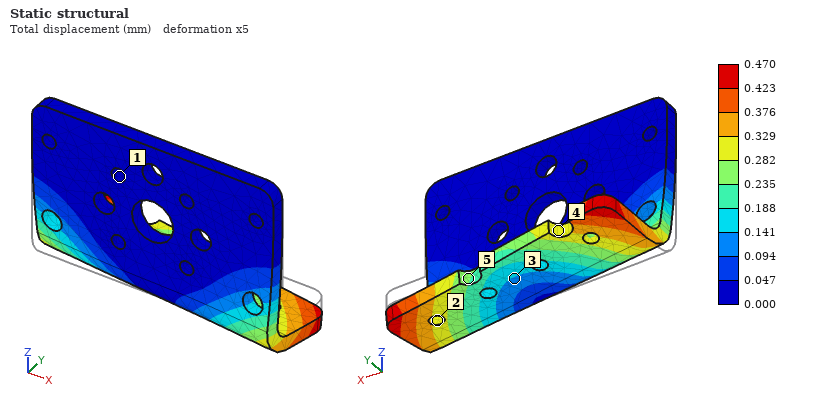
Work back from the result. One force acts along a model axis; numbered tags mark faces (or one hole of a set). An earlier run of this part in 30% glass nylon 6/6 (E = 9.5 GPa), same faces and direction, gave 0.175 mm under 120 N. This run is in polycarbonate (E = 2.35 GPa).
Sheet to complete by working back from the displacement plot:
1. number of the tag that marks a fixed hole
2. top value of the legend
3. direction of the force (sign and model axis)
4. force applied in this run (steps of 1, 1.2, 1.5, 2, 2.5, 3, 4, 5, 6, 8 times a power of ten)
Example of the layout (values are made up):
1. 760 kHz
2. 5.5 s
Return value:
1. 1
2. 0.470 mm
3. +X
4. 80 N
